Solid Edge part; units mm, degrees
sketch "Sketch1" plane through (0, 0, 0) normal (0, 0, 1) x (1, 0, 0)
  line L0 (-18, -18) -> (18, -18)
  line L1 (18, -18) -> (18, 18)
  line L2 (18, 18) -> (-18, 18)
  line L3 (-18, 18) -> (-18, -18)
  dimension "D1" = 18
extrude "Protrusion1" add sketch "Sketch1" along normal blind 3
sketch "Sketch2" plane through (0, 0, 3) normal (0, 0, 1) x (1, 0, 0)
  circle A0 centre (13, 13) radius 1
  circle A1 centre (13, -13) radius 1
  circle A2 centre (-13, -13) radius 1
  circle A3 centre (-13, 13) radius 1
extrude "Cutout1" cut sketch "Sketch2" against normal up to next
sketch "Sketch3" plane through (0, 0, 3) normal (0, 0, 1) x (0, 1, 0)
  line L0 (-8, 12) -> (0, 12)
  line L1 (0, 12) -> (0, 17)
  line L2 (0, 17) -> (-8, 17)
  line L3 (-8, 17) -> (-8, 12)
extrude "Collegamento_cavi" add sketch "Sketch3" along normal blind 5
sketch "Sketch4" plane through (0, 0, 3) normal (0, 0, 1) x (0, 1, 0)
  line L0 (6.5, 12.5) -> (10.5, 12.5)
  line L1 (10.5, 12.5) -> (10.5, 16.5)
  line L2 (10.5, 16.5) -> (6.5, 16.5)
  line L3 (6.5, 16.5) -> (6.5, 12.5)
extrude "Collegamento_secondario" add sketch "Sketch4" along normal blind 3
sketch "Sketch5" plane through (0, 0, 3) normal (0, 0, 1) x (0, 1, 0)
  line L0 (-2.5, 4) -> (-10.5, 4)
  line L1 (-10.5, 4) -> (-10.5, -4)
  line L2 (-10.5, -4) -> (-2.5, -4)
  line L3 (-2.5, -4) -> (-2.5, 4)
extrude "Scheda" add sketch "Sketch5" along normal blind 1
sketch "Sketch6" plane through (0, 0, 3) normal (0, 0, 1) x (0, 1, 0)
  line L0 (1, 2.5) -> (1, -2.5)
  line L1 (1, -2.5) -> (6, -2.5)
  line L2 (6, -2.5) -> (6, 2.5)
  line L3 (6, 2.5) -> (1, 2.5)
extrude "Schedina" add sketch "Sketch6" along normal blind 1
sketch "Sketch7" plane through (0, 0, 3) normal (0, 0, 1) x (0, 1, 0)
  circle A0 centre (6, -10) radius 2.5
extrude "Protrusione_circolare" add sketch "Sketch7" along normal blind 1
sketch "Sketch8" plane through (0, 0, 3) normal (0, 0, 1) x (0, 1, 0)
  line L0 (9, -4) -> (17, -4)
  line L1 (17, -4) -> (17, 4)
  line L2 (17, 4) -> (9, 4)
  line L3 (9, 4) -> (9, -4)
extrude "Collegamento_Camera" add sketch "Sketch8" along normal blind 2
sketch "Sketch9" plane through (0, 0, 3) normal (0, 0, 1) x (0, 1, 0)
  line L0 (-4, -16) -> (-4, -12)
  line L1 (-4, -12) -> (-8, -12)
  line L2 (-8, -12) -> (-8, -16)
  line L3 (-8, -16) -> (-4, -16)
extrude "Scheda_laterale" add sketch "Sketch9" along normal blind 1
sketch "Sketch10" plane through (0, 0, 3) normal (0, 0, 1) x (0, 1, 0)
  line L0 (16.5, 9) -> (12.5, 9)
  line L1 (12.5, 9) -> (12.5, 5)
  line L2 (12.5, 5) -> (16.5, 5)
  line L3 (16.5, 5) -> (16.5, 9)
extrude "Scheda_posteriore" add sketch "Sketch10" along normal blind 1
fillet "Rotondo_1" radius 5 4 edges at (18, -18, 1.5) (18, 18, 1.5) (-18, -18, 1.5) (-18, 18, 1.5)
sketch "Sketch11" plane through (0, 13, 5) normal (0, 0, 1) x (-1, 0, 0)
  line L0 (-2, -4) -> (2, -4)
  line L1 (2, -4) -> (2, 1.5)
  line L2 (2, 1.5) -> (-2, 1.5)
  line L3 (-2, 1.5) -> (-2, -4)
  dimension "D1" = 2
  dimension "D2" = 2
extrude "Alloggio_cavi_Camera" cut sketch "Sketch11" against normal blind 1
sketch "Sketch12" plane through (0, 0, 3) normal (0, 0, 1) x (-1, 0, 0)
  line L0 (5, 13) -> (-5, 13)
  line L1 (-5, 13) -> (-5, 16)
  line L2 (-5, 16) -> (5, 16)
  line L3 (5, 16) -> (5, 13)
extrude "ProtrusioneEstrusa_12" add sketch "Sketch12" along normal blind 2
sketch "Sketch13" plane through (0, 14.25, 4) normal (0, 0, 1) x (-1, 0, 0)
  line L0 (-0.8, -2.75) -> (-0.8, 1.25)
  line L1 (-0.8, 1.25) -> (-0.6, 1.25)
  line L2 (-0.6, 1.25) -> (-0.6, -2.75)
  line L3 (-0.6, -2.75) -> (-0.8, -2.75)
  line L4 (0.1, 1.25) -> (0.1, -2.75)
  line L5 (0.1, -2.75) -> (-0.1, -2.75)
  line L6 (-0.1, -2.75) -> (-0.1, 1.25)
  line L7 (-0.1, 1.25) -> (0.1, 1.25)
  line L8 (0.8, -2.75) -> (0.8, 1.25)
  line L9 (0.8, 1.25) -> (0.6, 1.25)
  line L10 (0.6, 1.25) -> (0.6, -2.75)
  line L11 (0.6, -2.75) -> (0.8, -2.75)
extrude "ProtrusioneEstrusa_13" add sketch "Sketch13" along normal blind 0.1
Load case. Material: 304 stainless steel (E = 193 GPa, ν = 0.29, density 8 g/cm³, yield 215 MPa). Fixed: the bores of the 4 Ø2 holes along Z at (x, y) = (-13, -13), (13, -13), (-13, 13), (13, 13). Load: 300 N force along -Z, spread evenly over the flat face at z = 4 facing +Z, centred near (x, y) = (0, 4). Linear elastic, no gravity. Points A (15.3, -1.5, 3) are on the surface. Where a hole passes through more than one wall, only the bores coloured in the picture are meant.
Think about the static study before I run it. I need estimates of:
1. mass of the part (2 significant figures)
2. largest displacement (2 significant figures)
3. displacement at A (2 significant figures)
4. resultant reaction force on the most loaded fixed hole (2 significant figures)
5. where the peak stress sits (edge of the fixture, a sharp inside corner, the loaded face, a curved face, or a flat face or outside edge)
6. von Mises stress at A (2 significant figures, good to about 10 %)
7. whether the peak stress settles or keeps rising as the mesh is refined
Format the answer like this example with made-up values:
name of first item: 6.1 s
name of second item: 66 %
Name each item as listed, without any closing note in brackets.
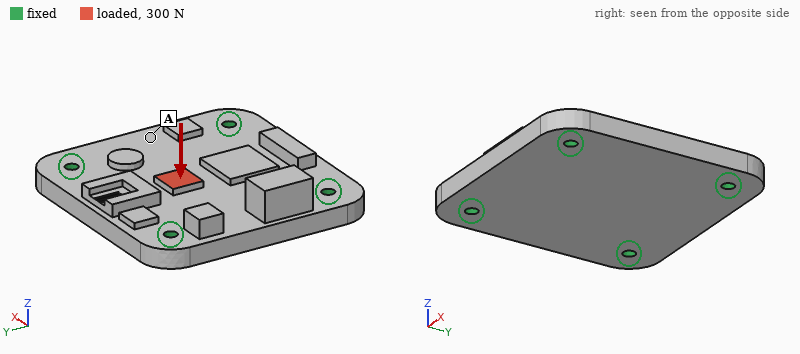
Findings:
mass of the part: 35 g
largest displacement: 5.1 µm
displacement at A: 1.1 µm
resultant reaction force on the most loaded fixed hole: 100 N
where the peak stress sits: edge of the fixture
von Mises stress at A: 8.2 MPa
whether the peak stress settles or keeps rising as the mesh is refined: keeps rising
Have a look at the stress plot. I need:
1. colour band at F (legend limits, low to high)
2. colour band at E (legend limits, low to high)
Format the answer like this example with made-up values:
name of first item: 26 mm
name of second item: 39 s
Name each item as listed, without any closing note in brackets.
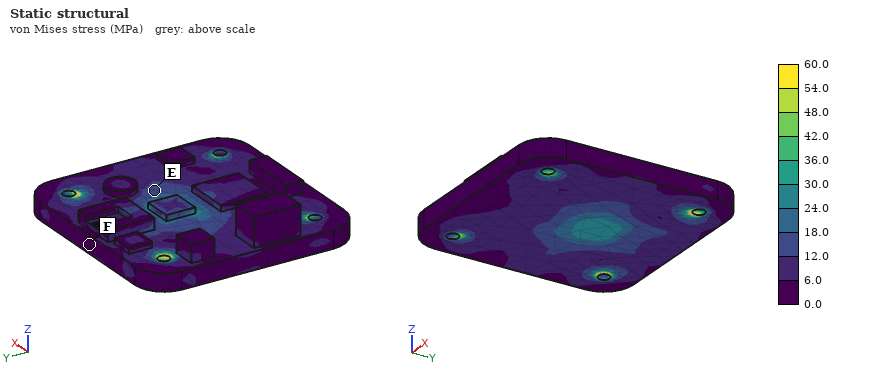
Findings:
colour band at F: 0.0 to 6.0 MPa
colour band at E: 12.0 to 18.0 MPa
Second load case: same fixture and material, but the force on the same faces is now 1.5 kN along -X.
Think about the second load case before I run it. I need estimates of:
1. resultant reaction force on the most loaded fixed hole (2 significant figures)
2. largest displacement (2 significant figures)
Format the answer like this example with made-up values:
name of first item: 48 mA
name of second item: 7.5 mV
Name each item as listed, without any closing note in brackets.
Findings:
resultant reaction force on the most loaded fixed hole: 500 N
largest displacement: 6.2 µm
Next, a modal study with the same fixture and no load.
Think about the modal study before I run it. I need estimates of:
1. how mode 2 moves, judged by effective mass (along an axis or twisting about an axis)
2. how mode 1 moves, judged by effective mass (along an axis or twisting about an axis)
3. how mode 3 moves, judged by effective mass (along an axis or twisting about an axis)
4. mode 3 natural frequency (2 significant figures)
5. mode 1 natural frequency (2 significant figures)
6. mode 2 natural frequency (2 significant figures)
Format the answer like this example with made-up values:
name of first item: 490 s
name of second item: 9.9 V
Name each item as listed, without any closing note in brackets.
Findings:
how mode 2 moves, judged by effective mass: twisting about Y
how mode 1 moves, judged by effective mass: along Z
how mode 3 moves, judged by effective mass: twisting about X
mode 3 natural frequency: 21 kHz
mode 1 natural frequency: 14 kHz
mode 2 natural frequency: 19 kHz
